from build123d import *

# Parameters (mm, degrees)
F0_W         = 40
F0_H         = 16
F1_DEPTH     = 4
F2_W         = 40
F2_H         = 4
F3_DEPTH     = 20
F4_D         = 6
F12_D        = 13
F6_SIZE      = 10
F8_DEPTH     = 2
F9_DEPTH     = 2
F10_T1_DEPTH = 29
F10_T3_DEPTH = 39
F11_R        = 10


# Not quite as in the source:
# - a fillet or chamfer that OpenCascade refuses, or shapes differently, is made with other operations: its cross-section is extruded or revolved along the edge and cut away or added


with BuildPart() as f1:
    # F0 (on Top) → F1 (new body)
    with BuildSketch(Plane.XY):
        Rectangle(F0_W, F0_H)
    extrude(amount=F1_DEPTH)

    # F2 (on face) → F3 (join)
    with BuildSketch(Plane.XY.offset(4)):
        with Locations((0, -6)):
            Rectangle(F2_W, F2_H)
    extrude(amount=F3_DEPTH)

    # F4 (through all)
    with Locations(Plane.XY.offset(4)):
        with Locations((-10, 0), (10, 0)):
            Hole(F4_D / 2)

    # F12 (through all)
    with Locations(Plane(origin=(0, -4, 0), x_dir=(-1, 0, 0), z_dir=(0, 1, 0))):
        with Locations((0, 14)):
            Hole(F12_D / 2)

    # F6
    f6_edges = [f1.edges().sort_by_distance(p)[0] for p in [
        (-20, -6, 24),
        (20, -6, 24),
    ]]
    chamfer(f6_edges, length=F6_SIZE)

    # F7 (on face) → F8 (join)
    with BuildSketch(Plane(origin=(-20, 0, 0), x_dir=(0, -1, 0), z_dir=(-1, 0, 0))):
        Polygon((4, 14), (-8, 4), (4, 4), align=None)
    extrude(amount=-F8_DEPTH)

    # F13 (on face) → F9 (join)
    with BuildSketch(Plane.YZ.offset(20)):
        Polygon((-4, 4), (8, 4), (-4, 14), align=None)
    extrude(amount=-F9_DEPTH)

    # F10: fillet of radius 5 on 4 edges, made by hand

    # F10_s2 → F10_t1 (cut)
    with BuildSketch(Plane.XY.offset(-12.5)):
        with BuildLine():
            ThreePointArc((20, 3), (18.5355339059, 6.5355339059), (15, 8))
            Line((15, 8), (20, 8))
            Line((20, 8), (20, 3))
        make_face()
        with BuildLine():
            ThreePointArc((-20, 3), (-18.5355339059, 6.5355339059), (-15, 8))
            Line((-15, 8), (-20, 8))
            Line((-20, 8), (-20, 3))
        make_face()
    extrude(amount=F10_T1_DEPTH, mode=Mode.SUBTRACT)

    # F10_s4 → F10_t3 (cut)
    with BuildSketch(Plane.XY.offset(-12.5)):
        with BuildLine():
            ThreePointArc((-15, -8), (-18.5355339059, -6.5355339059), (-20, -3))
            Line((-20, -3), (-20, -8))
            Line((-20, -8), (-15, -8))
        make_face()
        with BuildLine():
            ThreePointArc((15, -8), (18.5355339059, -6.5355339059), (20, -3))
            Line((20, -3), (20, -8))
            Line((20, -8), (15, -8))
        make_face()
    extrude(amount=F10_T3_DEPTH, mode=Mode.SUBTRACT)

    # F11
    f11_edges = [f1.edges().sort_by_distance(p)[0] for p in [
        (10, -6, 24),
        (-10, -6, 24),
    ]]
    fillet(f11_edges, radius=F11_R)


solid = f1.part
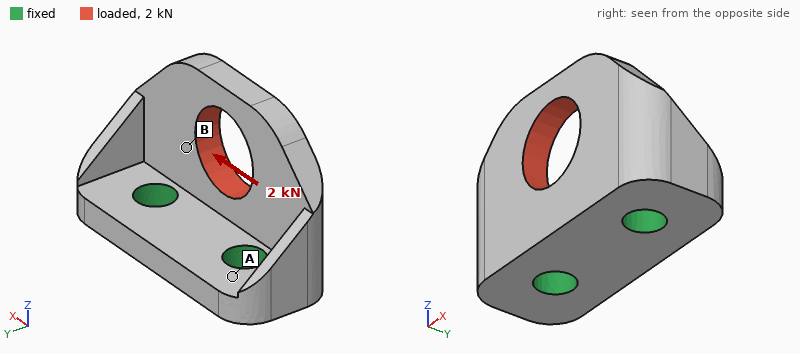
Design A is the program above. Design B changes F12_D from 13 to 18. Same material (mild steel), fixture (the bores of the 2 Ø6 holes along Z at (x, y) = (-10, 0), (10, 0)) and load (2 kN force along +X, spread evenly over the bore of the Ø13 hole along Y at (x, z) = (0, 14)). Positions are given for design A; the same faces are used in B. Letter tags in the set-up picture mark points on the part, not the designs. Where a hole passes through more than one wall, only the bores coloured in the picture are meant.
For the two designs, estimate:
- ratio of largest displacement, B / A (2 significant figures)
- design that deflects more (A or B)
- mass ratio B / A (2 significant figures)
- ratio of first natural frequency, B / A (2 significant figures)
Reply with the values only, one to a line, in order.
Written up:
2.0
B
0.89
1.1
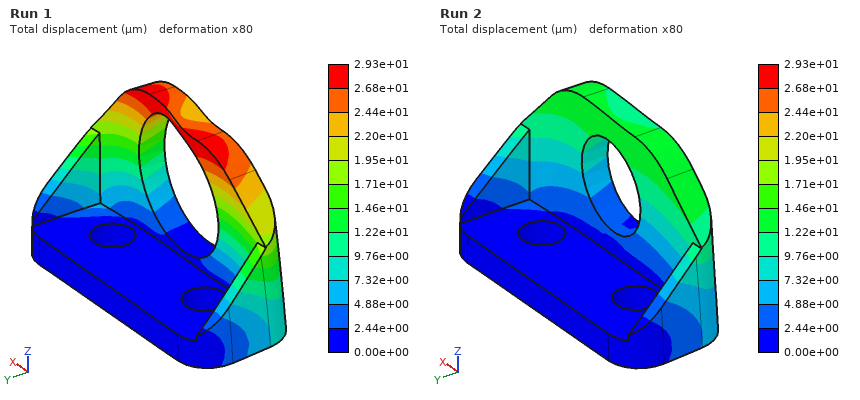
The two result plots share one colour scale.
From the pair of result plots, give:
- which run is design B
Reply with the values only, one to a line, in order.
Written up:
Run 1
